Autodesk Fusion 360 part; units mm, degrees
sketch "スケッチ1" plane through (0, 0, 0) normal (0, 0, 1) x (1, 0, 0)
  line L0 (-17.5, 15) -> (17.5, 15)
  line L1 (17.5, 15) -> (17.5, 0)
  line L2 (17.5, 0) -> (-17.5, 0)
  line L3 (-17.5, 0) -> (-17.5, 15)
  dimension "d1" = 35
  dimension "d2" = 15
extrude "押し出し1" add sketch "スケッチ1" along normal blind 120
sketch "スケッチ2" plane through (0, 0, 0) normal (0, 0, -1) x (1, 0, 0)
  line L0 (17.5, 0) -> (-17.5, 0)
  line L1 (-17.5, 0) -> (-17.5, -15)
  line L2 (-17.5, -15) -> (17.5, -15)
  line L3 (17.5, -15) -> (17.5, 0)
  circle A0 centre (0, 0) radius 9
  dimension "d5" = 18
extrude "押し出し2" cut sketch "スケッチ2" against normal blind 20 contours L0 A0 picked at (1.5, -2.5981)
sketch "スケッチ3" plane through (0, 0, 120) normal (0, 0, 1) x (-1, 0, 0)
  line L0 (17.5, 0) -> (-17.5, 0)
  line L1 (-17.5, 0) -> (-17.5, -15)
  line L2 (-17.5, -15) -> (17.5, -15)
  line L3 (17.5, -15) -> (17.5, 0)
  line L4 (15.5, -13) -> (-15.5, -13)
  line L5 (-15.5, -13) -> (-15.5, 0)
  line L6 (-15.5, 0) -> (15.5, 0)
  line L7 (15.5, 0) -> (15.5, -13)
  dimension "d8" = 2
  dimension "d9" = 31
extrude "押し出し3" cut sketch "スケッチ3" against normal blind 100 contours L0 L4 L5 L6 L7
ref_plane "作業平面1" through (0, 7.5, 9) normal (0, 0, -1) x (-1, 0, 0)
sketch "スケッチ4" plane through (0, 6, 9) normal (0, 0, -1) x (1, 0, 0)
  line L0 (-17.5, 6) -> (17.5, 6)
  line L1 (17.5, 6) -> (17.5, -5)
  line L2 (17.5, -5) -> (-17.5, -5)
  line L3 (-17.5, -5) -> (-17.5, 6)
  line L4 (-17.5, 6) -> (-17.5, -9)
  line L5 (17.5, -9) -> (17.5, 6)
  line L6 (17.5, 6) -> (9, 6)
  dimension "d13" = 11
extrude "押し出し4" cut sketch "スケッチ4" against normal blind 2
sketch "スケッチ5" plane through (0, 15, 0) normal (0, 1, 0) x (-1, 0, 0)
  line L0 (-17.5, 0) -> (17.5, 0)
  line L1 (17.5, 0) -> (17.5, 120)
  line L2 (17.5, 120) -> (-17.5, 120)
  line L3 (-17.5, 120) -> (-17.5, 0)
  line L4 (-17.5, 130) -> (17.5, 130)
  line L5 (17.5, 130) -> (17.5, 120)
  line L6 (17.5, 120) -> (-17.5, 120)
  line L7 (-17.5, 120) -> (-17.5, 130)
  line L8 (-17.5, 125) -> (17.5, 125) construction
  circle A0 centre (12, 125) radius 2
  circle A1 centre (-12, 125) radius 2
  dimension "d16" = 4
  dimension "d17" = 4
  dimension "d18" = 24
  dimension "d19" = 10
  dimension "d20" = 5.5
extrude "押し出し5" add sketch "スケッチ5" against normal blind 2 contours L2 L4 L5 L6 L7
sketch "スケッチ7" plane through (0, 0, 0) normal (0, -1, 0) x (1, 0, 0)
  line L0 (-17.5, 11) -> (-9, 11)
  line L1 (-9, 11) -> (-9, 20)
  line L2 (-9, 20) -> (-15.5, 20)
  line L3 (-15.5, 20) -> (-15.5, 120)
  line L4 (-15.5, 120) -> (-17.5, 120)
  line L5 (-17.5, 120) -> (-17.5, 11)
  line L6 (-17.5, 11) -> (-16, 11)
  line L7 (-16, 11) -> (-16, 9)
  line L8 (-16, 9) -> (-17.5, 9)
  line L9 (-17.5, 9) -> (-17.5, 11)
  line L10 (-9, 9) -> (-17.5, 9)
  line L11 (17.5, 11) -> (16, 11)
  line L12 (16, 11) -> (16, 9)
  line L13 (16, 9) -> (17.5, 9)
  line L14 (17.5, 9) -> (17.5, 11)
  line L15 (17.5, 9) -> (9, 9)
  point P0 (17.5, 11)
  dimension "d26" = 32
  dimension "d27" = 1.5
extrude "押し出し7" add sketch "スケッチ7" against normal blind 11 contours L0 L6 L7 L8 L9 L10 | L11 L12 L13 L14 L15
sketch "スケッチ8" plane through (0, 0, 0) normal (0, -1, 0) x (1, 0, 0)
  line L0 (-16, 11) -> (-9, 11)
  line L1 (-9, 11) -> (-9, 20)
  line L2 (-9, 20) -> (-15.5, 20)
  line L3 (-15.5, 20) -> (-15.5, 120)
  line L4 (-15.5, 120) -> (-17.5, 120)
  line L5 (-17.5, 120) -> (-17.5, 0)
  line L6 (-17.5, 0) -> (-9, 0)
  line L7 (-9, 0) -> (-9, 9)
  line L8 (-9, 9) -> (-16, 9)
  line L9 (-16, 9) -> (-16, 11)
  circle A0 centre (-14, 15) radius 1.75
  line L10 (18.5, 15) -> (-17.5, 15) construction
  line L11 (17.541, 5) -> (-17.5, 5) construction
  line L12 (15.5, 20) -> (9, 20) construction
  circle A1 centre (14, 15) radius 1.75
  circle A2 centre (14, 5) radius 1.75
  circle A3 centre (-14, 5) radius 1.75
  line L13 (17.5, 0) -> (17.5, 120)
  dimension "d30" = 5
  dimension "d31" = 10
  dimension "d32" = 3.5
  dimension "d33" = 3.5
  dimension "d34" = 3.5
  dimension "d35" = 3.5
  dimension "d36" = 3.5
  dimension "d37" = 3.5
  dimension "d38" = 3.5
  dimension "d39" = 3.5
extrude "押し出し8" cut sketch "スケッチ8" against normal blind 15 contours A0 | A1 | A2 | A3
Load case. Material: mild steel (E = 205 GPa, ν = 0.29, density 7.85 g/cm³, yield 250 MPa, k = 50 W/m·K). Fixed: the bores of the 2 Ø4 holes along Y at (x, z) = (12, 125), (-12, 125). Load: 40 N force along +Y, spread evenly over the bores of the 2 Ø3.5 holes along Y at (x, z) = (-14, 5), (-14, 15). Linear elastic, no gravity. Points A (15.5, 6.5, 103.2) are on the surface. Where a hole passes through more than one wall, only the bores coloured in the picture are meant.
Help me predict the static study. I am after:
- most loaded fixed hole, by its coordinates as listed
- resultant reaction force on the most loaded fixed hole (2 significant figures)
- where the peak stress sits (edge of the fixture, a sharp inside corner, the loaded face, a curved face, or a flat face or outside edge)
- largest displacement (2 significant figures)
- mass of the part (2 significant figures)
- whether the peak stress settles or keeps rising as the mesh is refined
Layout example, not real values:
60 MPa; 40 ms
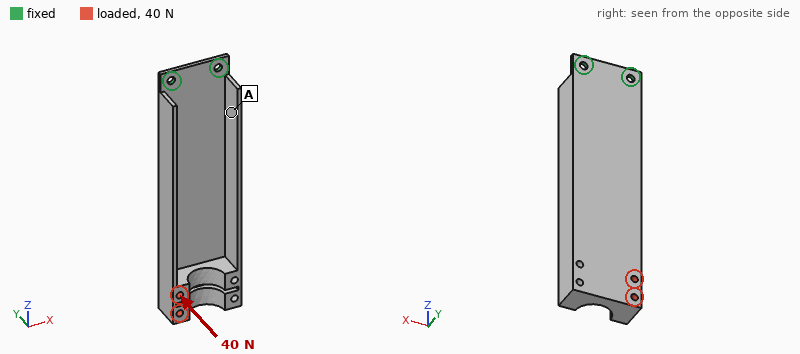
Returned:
(-12, 125); 81 N; edge of the fixture; 1.00 mm; 160 g; keeps rising
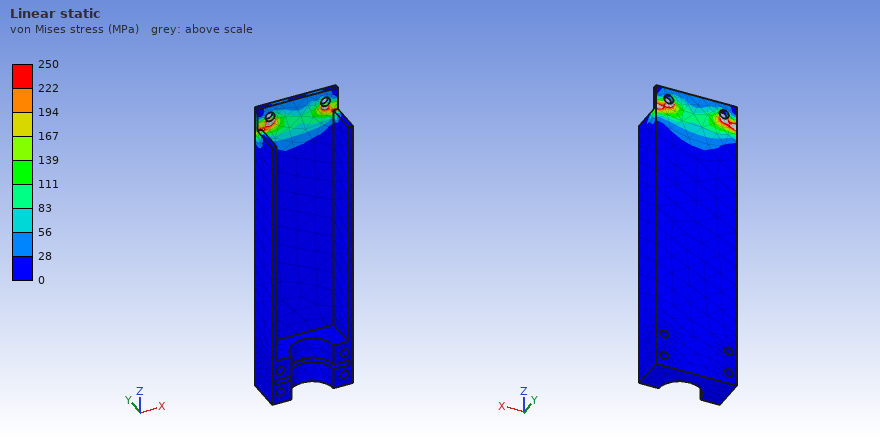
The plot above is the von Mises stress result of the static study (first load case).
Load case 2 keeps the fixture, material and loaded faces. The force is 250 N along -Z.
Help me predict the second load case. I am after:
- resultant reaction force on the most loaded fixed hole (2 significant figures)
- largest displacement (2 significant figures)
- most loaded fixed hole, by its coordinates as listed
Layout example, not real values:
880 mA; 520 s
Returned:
260 N; 0.36 mm; (-12, 125)
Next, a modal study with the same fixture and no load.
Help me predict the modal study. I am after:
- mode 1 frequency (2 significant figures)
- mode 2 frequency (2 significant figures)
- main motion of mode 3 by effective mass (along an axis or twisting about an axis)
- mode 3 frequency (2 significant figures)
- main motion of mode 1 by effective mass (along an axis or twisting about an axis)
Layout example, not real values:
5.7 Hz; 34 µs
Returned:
120 Hz; 660 Hz; along X; 1100 Hz; along Y
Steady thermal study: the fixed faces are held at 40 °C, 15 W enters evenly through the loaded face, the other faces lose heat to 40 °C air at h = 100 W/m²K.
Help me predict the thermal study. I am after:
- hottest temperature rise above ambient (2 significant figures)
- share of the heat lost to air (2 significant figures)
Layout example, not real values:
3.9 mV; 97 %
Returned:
41 K; 100 %
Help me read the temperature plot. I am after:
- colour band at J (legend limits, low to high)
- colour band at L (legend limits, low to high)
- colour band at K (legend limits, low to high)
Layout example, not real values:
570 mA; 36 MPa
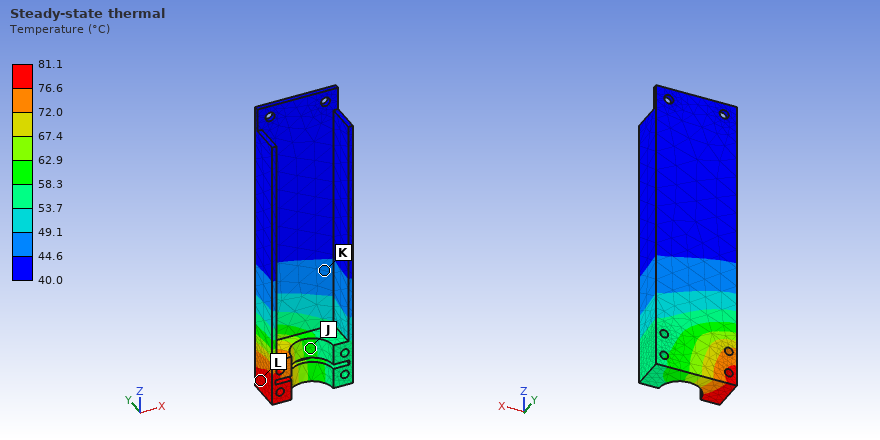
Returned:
58.3 to 62.9 °C; 76.6 to 81.1 °C; 44.6 to 49.1 °C
